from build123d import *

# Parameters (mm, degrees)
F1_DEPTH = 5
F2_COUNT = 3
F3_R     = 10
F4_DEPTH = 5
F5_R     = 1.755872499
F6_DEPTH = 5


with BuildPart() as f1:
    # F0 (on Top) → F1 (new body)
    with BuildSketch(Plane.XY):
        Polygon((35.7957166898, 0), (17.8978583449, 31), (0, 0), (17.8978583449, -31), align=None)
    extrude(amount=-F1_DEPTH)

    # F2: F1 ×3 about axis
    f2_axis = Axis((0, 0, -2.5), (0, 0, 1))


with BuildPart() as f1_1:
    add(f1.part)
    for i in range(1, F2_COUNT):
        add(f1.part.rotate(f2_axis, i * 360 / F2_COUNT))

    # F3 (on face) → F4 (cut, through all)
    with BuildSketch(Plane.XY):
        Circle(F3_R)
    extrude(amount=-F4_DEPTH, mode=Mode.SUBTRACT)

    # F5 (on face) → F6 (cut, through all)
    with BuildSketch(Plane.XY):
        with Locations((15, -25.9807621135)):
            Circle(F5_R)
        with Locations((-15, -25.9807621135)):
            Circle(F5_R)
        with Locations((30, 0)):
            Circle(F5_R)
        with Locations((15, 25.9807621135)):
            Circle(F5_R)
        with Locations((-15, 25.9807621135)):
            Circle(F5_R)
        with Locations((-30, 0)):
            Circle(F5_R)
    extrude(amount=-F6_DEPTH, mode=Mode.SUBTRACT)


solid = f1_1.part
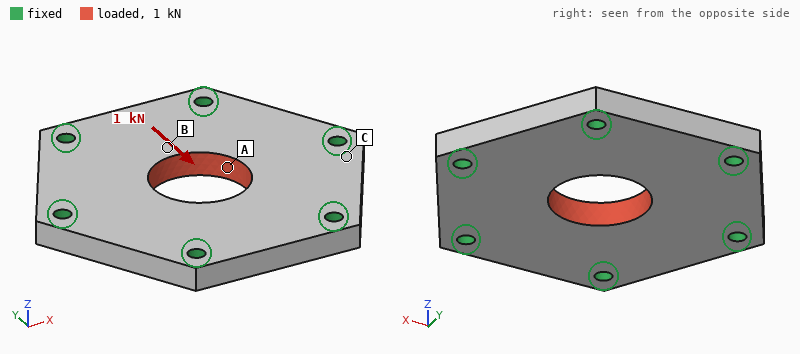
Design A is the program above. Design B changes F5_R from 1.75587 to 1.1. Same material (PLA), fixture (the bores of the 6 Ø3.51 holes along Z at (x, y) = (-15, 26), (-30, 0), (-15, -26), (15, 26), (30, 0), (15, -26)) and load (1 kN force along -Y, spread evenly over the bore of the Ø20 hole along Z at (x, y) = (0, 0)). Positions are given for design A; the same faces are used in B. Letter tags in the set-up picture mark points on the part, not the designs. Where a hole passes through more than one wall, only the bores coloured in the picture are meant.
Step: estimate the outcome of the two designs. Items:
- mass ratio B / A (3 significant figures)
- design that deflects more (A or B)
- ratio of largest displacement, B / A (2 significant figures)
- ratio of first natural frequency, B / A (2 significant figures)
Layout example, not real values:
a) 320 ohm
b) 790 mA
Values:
a) 1.01
b) B
c) 1.1
d) 0.90
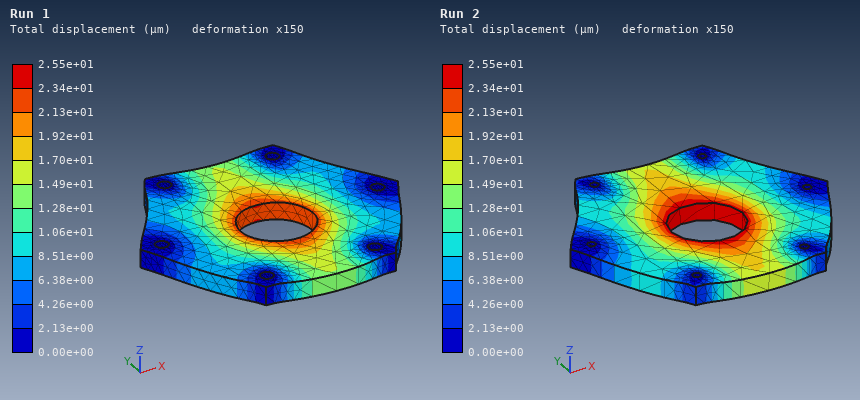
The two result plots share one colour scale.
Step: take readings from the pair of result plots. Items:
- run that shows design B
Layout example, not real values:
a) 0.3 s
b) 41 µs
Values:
a) Run 2
